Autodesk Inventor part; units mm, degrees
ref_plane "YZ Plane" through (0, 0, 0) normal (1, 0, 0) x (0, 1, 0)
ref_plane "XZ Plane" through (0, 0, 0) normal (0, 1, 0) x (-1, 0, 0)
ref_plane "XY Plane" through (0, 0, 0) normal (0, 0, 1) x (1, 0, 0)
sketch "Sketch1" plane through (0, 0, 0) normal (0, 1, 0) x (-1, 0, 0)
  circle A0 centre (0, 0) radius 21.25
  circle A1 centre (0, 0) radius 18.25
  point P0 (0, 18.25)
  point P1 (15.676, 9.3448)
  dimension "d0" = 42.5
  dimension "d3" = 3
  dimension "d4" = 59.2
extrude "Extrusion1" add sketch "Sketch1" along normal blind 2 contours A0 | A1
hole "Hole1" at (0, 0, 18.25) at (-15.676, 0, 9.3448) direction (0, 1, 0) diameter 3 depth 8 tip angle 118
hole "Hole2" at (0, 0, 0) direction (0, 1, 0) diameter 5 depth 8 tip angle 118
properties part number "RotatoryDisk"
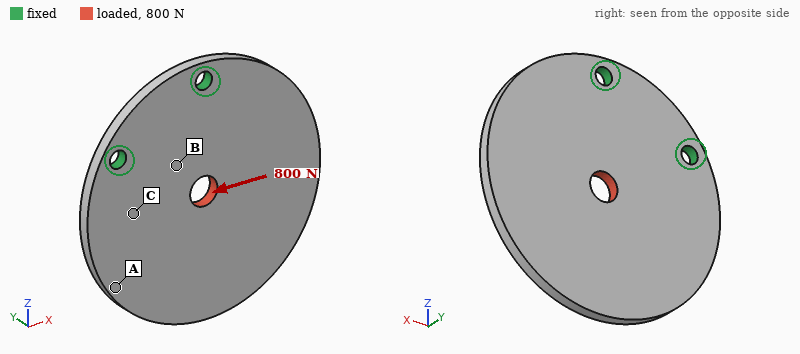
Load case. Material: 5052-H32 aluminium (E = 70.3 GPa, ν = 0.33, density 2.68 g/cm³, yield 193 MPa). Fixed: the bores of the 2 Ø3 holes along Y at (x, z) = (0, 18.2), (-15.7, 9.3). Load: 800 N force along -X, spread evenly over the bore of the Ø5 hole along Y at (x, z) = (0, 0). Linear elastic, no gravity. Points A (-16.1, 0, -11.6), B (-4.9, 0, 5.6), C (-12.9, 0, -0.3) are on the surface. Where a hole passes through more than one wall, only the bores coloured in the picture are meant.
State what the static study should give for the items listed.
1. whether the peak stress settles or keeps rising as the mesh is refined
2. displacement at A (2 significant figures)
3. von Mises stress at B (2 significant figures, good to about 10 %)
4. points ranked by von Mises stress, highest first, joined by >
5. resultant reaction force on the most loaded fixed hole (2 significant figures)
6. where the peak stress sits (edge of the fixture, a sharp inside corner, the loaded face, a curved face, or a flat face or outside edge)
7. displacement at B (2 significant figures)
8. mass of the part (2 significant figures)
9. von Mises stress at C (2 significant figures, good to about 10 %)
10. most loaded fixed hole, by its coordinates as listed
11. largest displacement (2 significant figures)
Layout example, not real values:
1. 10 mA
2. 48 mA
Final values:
1. keeps rising
2. 18 µm
3. 37 MPa
4. B > C > A
5. 830 N
6. edge of the fixture
7. 7.2 µm
8. 7.4 g
9. 19 MPa
10. (-15.7, 9.3)
11. 24 µm
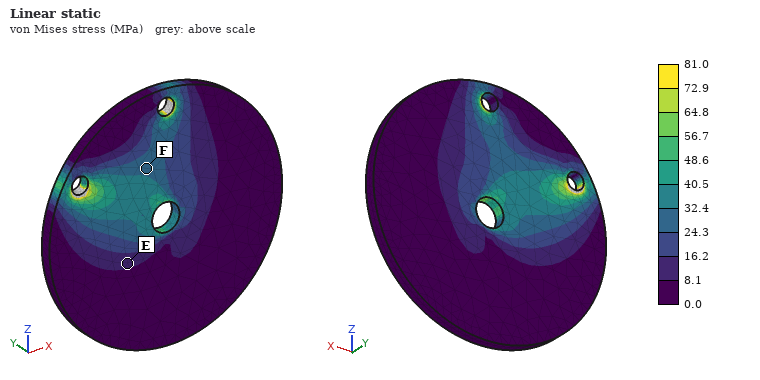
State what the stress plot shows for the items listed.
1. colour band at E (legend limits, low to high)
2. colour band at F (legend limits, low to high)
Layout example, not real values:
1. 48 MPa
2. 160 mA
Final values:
1. 8.1 to 16.2 MPa
2. 24.3 to 32.4 MPa
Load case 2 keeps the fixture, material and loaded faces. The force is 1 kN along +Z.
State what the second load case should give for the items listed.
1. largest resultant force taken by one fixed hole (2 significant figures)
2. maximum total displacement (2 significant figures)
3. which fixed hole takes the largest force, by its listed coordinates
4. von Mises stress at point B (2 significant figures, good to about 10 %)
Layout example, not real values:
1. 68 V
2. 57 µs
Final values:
1. 870 N
2. 18 µm
3. (0, 18.2)
4. 26 MPa
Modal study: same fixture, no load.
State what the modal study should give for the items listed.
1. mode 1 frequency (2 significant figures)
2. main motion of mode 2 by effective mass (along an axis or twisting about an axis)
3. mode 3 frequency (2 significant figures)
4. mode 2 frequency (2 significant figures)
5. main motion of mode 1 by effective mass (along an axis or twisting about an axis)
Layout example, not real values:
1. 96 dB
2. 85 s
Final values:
1. 1400 Hz
2. twisting about Z
3. 6600 Hz
4. 3100 Hz
5. along Y
